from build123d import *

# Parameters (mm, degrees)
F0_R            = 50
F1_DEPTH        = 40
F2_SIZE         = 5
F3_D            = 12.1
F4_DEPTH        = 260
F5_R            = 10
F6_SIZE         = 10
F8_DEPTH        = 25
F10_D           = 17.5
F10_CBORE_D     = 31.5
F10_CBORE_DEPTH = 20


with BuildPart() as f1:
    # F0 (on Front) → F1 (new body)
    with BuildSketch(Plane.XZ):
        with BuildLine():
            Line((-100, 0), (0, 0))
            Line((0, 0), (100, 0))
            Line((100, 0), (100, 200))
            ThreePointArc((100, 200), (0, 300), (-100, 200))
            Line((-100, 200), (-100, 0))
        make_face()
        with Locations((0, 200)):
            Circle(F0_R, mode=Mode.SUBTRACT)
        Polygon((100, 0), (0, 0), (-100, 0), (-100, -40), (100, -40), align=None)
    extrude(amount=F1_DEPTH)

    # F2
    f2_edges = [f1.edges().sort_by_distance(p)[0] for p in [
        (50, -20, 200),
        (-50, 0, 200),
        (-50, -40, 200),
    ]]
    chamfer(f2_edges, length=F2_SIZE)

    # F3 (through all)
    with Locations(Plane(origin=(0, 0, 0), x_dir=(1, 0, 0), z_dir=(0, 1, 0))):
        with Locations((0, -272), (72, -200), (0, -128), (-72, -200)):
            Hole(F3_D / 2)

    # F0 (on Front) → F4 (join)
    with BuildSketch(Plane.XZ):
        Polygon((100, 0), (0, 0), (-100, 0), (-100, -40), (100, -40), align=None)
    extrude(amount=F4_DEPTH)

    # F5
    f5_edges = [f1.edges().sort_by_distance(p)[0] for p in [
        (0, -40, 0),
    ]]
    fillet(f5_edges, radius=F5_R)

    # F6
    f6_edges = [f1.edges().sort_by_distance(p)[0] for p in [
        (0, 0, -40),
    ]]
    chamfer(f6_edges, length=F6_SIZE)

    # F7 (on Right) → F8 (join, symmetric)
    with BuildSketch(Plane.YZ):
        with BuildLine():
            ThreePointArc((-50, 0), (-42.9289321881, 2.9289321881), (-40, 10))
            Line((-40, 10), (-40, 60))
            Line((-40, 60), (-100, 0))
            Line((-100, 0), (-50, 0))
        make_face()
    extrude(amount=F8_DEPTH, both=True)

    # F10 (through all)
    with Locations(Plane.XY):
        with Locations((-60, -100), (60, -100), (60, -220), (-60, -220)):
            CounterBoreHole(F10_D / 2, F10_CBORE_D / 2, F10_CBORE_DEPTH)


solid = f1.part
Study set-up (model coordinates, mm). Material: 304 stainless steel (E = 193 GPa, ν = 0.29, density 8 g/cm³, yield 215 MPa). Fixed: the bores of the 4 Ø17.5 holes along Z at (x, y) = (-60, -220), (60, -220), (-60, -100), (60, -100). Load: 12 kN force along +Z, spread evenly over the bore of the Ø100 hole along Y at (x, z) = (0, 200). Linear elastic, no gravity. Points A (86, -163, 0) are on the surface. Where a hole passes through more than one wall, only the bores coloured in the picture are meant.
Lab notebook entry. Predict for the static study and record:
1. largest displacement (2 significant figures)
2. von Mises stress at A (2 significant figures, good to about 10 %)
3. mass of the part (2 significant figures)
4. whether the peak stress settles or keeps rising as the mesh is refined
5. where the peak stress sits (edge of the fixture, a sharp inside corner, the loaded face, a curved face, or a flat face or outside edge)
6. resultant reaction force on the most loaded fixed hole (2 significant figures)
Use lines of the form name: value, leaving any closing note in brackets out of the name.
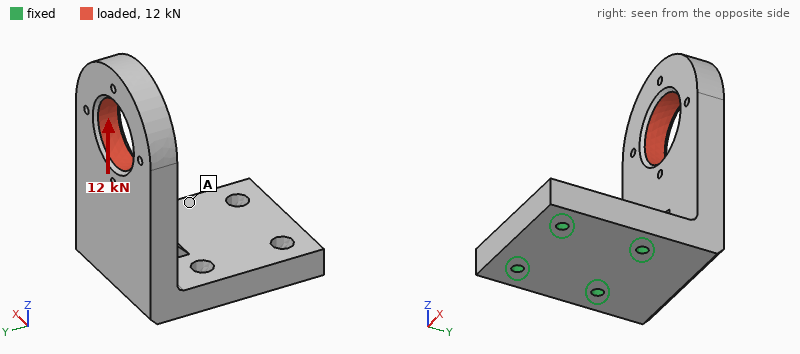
largest displacement: 87 µm
von Mises stress at A: 4.2 MPa
mass of the part: 32 kg
whether the peak stress settles or keeps rising as the mesh is refined: keeps rising
where the peak stress sits: edge of the fixture
resultant reaction force on the most loaded fixed hole: 9.9 kN
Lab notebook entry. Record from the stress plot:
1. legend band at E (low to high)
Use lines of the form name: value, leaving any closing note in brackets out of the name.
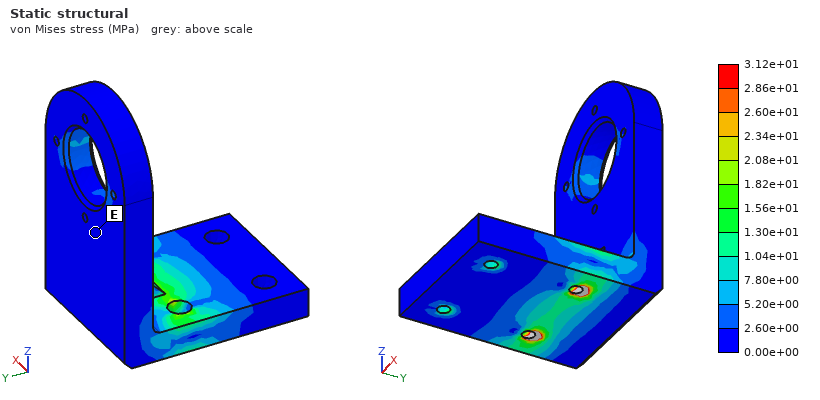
legend band at E: 0.00e+00 to 2.60e+00 MPa
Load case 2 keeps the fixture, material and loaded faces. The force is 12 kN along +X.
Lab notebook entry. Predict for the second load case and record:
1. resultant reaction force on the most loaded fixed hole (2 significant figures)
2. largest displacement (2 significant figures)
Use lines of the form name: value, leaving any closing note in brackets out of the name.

resultant reaction force on the most loaded fixed hole: 25 kN
largest displacement: 0.12 mm
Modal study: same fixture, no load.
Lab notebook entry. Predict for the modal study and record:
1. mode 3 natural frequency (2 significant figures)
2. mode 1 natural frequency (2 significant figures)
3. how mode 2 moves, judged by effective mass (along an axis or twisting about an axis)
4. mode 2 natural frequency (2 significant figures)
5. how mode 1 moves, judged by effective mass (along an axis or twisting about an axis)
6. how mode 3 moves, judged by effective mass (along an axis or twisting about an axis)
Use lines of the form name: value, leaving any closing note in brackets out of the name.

mode 3 natural frequency: 1100 Hz
mode 1 natural frequency: 310 Hz
how mode 2 moves, judged by effective mass: along X
mode 2 natural frequency: 610 Hz
how mode 1 moves, judged by effective mass: along Y
how mode 3 moves, judged by effective mass: along Z
